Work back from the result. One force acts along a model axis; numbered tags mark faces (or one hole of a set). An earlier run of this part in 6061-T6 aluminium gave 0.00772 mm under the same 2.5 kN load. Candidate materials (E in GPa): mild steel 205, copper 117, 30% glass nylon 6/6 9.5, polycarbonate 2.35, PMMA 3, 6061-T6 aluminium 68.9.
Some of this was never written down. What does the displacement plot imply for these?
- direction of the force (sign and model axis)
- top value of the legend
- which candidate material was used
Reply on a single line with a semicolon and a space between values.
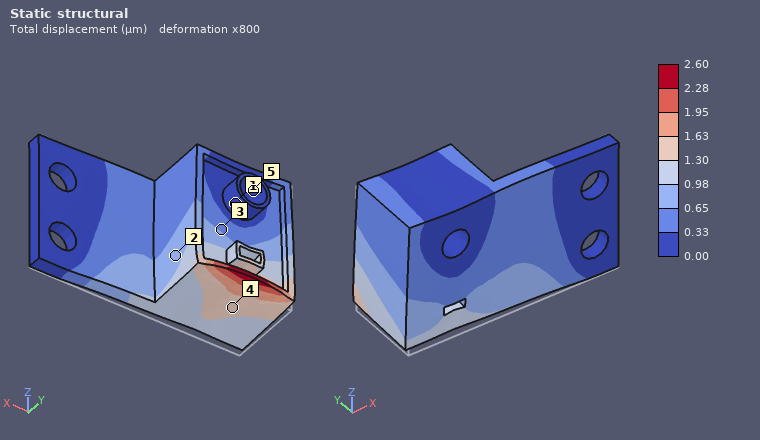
+Z; 2.60 µm; mild steel
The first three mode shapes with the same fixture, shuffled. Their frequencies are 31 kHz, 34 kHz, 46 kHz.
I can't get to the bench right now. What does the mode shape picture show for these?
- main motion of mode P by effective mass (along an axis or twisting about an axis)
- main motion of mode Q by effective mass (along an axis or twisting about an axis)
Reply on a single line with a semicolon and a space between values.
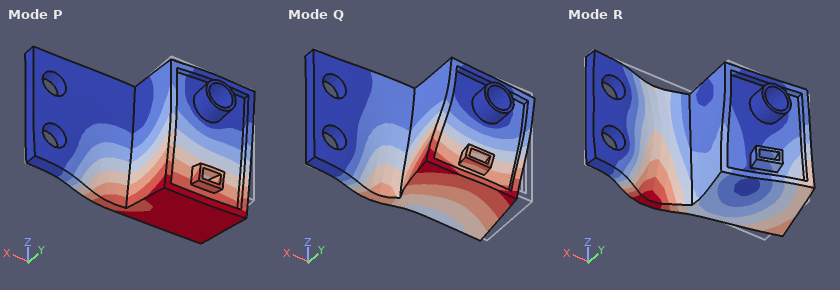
along Y; along X
